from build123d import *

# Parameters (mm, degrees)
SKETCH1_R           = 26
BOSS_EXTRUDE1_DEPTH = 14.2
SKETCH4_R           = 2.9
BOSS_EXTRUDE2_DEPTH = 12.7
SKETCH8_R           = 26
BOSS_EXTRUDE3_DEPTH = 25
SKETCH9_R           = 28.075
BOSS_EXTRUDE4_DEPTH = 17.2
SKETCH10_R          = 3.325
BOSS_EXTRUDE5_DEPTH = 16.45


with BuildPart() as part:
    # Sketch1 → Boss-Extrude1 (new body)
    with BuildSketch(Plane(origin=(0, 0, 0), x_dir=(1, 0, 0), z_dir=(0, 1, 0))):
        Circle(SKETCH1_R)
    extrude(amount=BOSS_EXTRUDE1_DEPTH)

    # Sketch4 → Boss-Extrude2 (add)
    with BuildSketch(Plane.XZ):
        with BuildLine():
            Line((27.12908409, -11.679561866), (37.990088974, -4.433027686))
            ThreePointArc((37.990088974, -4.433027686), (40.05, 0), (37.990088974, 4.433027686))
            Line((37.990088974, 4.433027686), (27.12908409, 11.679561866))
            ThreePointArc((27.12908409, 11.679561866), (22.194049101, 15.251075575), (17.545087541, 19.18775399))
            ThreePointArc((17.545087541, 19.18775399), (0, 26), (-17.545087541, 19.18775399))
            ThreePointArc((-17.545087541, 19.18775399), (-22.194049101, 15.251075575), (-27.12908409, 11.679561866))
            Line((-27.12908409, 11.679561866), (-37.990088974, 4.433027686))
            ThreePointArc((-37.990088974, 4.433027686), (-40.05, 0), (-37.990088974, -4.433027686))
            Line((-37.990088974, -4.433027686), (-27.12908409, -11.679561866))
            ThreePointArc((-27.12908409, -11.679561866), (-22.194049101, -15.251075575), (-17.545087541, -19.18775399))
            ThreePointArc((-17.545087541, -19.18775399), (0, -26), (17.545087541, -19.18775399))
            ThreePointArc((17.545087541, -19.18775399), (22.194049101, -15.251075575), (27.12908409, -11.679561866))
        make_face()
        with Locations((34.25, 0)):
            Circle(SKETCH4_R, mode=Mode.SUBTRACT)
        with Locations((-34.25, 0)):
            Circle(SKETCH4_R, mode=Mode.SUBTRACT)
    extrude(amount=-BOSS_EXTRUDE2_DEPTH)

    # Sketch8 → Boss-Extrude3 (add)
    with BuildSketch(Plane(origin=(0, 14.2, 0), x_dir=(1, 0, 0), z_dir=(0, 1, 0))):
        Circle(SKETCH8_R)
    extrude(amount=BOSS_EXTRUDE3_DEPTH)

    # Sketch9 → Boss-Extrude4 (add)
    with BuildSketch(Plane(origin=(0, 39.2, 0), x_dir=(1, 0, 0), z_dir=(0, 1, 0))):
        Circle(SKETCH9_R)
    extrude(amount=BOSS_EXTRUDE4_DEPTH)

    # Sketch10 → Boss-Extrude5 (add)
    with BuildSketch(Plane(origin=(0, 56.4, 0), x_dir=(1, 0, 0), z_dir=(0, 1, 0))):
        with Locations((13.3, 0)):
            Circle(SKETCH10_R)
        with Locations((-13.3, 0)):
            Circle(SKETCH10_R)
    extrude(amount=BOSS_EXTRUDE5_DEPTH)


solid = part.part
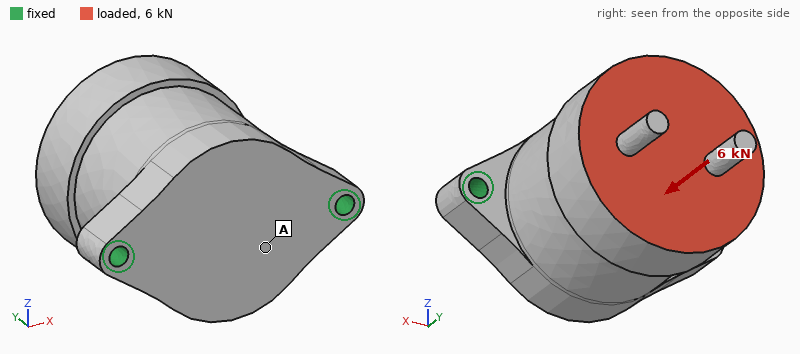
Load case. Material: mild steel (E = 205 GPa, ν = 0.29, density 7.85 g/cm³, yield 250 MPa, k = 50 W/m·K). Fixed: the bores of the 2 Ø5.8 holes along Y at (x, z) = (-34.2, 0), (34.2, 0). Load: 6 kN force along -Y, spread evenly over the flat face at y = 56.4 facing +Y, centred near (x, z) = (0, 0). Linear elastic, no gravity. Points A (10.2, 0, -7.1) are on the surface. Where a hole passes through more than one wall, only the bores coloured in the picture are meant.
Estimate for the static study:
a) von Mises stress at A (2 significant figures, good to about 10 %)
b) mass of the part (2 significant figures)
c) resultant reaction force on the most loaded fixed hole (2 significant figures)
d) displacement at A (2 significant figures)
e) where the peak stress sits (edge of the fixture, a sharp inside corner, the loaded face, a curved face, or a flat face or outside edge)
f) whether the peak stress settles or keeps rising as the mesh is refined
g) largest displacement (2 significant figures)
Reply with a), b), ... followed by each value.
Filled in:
a) 7.6 MPa
b) 1.0 kg
c) 3.2 kN
d) 3.5 µm
e) edge of the fixture
f) keeps rising
g) 4.1 µm
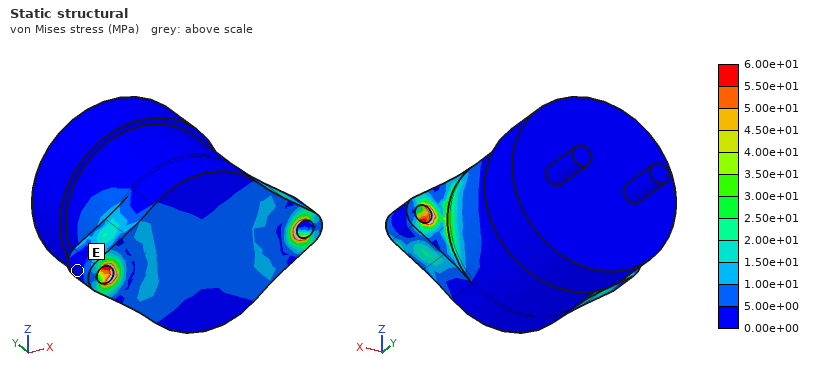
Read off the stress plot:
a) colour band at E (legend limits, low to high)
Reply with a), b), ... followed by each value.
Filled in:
a) 0.00e+00 to 5.00e+00 MPa
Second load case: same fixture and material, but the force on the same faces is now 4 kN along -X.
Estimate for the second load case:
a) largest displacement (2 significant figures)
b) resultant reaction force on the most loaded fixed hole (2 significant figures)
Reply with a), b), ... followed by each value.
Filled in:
a) 12 µm
b) 3.9 kN
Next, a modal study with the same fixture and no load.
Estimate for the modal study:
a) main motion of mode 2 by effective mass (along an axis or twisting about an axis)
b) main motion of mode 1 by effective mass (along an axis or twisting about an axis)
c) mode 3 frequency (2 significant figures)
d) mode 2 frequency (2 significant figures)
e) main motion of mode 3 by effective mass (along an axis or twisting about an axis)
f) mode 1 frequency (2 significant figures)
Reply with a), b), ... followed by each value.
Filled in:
a) along X
b) along Z
c) 6500 Hz
d) 5600 Hz
e) along Y
f) 1700 Hz
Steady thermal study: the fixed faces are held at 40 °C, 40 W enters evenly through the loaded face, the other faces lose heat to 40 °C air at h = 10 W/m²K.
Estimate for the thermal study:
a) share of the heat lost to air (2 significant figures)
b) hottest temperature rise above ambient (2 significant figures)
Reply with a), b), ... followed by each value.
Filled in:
a) 8.6 %
b) 37 K
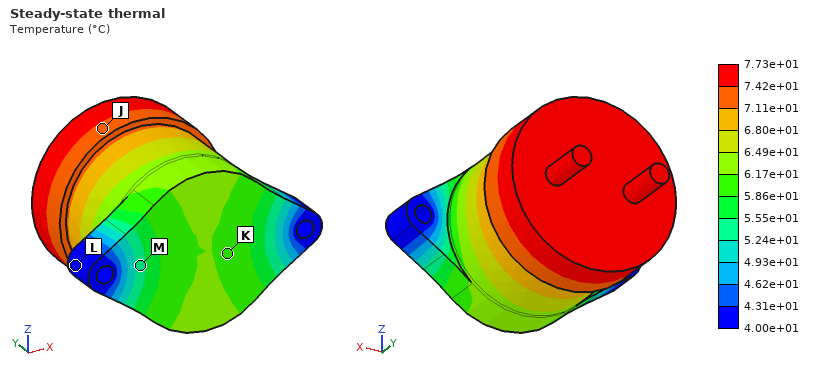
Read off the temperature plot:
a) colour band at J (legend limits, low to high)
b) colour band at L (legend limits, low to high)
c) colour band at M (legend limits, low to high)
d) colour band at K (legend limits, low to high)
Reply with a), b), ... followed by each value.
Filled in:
a) 7.11e+01 to 7.42e+01 °C
b) 4.00e+01 to 4.31e+01 °C
c) 5.24e+01 to 5.55e+01 °C
d) 5.86e+01 to 6.17e+01 °C
